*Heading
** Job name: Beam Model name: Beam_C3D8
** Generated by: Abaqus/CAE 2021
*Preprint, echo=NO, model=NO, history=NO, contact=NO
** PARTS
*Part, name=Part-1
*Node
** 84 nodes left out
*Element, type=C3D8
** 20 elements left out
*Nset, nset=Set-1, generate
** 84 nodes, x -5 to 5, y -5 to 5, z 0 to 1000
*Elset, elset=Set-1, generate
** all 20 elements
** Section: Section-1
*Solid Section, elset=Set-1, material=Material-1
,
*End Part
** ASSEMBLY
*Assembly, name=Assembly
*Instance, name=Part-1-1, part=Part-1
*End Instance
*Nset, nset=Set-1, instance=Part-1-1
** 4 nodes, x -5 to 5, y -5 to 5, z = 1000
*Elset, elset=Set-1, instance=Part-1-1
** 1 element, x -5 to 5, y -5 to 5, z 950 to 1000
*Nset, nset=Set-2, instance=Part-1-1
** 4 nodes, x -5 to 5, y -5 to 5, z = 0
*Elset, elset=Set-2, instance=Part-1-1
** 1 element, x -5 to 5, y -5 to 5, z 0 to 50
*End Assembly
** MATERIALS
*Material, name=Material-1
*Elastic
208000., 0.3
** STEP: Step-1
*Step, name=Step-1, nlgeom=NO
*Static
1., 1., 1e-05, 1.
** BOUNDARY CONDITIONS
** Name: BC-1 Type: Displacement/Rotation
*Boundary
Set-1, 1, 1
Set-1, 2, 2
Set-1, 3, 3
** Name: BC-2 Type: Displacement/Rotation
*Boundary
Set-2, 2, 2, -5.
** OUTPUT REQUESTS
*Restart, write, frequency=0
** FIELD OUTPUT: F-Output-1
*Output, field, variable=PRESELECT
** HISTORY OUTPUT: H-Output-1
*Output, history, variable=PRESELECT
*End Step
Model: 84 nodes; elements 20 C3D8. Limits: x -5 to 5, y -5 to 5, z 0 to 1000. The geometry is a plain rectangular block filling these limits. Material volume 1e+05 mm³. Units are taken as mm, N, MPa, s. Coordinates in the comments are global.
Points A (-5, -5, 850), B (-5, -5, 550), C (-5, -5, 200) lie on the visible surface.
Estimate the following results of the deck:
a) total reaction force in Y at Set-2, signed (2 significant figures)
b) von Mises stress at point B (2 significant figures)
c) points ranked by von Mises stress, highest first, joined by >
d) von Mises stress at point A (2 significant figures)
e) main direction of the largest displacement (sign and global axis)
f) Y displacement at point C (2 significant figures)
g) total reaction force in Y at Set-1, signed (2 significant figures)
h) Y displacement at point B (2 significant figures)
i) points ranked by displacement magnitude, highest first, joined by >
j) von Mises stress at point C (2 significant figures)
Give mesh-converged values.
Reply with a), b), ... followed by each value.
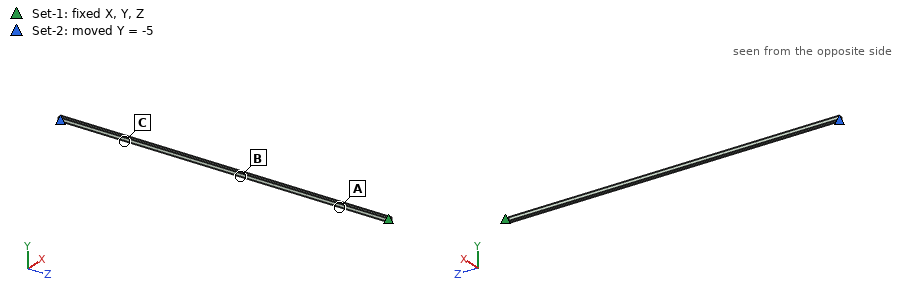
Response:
a) -2.6 N
b) 8.7 MPa
c) A > B > C
d) 13 MPa
e) -Y
f) -3.5 mm
g) 2.6 N
h) -1.3 mm
i) C > B > A
j) 3.2 MPa
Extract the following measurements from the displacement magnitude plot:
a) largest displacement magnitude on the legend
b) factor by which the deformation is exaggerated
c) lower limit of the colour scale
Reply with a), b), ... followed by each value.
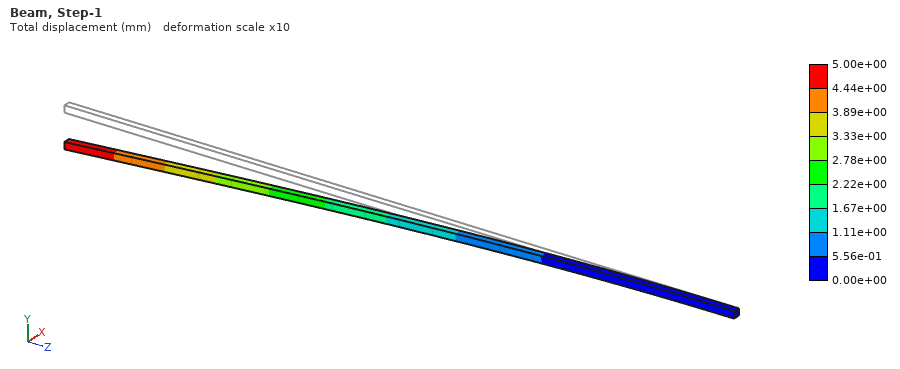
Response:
a) 5.00e+00 mm
b) 10
c) 0.00e+00 mm
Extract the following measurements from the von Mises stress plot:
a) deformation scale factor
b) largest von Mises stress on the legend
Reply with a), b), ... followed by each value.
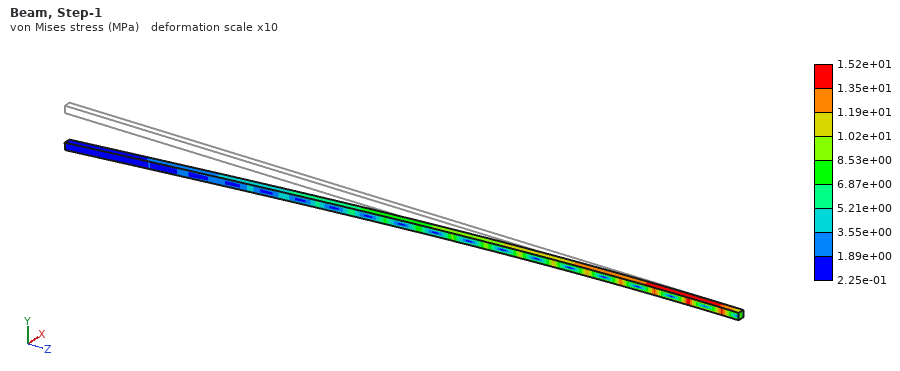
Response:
a) 10
b) 1.52e+01 MPa
